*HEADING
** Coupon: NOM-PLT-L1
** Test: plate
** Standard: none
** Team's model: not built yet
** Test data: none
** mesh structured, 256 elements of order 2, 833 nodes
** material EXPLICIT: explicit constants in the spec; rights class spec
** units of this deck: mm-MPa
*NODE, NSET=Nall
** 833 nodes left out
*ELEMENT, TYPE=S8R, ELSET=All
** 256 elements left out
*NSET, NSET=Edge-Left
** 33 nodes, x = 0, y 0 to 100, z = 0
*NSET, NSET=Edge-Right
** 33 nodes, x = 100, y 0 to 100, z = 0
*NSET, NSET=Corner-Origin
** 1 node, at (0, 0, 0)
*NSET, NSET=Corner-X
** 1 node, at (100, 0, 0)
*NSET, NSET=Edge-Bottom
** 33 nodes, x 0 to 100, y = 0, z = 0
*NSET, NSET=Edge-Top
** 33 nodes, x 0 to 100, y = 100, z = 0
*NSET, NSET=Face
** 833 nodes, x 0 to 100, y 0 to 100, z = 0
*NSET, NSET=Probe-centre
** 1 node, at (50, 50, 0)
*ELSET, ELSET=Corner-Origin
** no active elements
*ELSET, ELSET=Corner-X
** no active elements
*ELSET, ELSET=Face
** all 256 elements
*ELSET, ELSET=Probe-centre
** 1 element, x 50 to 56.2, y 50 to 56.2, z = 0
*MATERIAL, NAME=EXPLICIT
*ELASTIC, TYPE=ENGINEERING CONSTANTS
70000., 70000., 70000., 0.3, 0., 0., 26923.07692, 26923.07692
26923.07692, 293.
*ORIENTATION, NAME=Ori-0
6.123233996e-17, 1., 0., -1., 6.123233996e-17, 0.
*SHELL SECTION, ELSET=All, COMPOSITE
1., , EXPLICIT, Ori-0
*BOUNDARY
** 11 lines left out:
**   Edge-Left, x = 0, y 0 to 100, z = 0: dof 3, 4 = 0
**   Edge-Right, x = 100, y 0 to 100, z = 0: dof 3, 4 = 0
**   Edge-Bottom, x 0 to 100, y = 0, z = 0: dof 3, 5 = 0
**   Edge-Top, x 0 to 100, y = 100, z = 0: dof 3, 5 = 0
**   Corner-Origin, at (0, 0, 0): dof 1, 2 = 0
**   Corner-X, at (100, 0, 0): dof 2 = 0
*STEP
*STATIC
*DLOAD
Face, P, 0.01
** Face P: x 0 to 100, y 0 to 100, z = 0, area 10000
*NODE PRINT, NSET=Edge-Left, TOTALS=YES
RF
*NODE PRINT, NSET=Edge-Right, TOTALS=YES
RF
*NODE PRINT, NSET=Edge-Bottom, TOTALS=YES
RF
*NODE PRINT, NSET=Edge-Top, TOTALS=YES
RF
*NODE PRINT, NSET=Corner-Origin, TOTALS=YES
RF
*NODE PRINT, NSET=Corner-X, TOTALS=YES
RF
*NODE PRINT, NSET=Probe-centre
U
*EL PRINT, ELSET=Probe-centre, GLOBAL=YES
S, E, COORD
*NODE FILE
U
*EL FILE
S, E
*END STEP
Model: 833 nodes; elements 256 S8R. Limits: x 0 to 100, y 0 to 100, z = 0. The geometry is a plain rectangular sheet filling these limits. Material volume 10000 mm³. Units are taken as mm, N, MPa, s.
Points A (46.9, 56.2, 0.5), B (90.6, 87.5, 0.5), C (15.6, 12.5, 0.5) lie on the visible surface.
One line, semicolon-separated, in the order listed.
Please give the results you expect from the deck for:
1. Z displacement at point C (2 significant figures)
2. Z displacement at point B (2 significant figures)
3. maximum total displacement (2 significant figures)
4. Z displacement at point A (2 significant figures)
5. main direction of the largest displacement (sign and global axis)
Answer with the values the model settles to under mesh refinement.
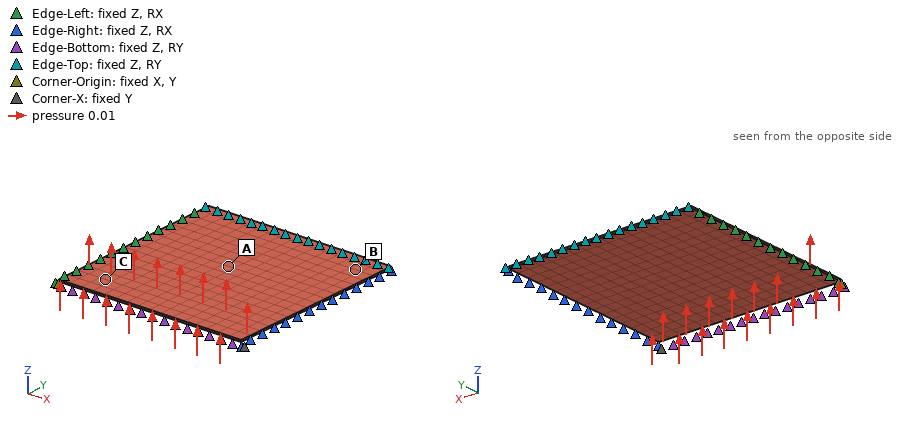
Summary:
0.13 mm; 0.079 mm; 0.63 mm; 0.62 mm; +Z
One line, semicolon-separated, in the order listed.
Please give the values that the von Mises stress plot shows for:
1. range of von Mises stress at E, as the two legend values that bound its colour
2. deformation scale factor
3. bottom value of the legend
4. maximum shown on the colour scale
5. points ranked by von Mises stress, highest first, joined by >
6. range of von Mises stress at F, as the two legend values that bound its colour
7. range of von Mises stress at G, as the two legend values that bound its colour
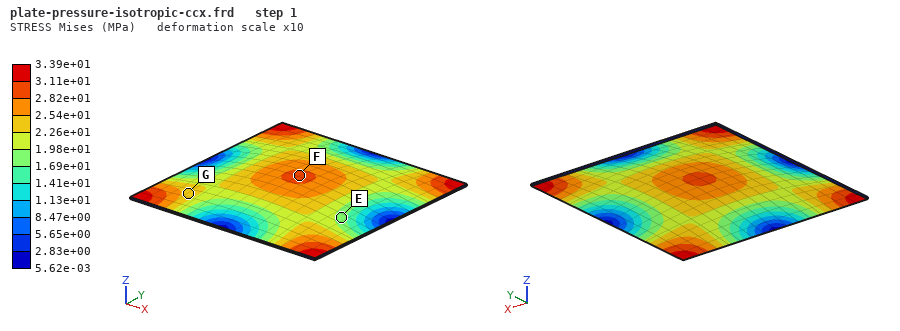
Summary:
1.69e+01 to 1.98e+01 MPa; 10; 5.62e-03 MPa; 3.39e+01 MPa; F > G > E; 2.82e+01 to 3.11e+01 MPa; 2.26e+01 to 2.54e+01 MPa
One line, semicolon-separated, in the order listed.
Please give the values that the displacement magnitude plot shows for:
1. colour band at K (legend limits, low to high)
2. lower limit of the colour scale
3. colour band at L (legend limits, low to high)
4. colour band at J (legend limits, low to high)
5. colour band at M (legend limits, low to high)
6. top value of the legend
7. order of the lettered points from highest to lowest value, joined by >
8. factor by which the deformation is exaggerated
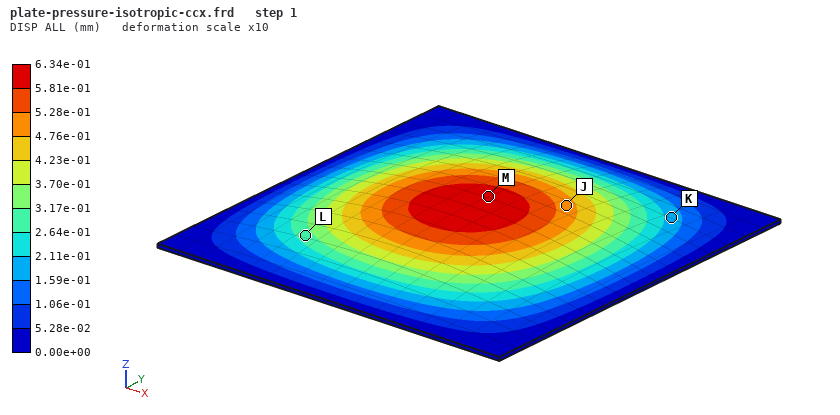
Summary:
1.59e-01 to 2.11e-01 mm; 0.00e+00 mm; 2.64e-01 to 3.17e-01 mm; 4.76e-01 to 5.28e-01 mm; 5.81e-01 to 6.34e-01 mm; 6.34e-01 mm; M > J > L > K; 10
